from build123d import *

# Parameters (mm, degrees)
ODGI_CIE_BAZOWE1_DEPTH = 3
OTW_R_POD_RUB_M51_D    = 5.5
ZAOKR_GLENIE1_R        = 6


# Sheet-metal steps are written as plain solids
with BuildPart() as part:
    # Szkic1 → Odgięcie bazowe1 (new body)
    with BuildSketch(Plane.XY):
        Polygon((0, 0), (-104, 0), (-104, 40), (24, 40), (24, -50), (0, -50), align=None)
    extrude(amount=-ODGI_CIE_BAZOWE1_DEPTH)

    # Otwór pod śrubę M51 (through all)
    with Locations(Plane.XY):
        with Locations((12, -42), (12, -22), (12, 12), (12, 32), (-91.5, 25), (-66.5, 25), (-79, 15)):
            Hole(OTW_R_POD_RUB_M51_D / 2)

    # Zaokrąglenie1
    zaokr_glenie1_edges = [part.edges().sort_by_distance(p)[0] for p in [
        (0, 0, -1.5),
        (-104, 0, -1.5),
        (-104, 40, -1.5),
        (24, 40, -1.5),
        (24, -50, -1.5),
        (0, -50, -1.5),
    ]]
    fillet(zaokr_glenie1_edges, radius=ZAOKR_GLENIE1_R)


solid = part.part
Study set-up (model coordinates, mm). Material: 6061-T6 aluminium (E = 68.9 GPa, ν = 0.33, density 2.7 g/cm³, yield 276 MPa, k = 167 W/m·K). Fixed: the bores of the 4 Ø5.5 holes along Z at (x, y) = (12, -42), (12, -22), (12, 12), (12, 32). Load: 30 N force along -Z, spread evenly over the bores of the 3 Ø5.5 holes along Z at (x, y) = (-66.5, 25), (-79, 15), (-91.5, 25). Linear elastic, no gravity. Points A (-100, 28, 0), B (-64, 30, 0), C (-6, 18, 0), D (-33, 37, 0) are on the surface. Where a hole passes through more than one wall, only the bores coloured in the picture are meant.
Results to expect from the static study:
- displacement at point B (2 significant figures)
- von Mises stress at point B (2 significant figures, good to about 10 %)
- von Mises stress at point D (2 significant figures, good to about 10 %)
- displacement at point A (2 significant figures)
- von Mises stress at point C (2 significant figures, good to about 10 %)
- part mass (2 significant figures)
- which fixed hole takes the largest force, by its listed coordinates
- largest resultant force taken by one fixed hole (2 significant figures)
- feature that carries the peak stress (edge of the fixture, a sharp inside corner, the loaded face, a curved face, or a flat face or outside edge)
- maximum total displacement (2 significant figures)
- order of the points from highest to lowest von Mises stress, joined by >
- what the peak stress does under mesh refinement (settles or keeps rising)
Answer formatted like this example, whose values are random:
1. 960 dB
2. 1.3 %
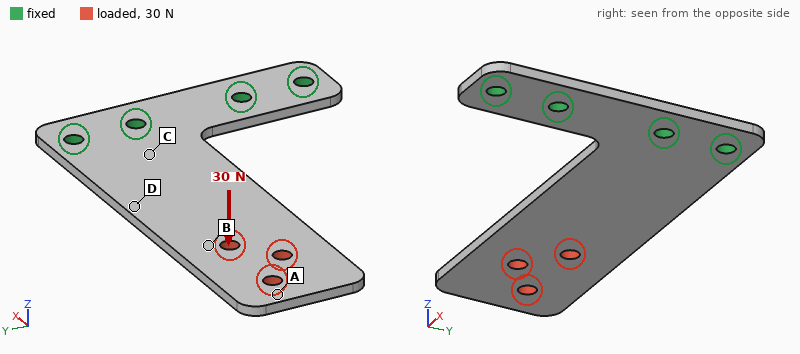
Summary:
1. 0.82 mm
2. 9.1 MPa
3. 23 MPa
4. 1.5 mm
5. 33 MPa
6. 50 g
7. (12, 12)
8. 29 N
9. edge of the fixture
10. 1.6 mm
11. C > D > B > A
12. keeps rising
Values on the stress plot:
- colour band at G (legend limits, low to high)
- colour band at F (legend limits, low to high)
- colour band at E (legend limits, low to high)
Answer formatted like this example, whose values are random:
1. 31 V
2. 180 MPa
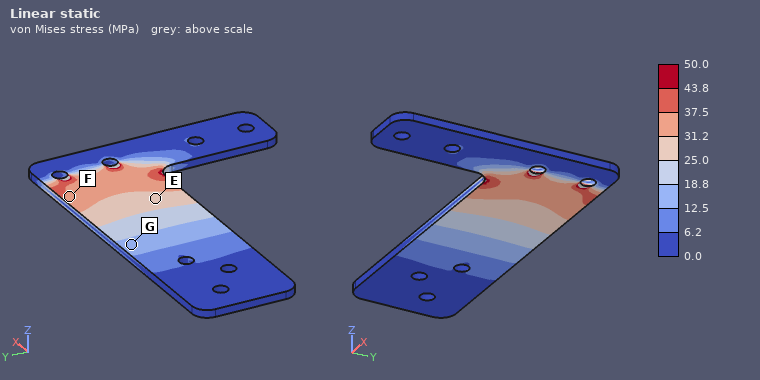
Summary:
1. 12.5 to 18.8 MPa
2. 31.2 to 37.5 MPa
3. 25.0 to 31.2 MPa
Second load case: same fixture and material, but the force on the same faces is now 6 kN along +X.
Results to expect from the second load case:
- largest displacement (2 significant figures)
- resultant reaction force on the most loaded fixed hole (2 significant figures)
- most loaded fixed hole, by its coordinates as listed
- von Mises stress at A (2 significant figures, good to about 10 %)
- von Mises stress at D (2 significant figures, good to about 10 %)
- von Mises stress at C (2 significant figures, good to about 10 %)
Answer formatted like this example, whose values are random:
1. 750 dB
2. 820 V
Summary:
1. 0.10 mm
2. 3.2 kN
3. (12, 32)
4. 23 MPa
5. 61 MPa
6. 47 MPa
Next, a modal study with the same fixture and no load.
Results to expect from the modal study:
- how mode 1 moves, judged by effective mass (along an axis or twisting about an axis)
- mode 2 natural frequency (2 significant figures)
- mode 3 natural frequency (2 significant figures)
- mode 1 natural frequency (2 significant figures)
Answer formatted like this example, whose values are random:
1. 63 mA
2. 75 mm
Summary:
1. along Z
2. 1100 Hz
3. 1200 Hz
4. 200 Hz
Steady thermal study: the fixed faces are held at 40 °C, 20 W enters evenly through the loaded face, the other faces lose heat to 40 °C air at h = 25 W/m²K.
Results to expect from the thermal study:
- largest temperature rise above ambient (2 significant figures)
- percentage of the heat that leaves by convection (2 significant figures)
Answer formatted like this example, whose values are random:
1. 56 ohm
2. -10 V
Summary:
1. 62 K
2. 42 %
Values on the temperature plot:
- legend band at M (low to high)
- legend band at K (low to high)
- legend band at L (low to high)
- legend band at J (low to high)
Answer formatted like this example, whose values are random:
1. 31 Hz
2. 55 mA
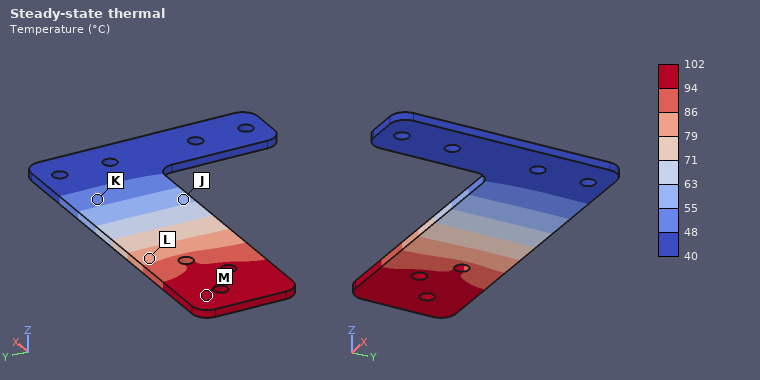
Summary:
1. 94 to 102 °C
2. 48 to 55 °C
3. 79 to 86 °C
4. 55 to 63 °C
